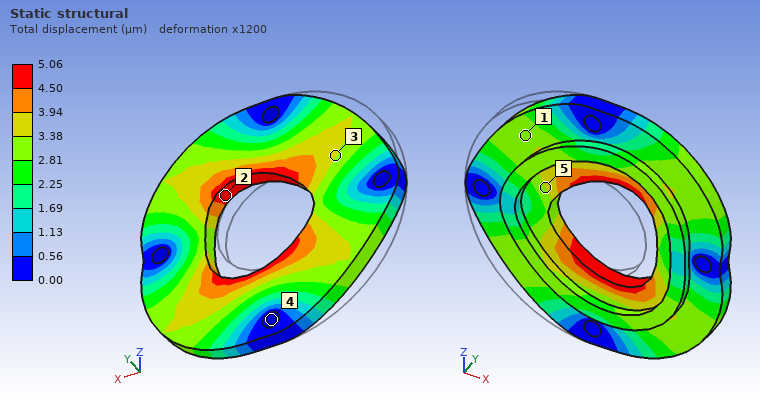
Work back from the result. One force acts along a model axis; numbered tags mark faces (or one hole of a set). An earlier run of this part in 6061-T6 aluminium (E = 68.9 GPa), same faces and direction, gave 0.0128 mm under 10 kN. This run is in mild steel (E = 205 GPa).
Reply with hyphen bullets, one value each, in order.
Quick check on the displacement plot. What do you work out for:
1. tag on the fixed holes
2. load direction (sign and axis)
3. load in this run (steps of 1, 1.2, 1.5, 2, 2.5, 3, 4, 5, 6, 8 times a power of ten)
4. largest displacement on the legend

- 4
- +X
- 12 kN
- 5.06 µm
